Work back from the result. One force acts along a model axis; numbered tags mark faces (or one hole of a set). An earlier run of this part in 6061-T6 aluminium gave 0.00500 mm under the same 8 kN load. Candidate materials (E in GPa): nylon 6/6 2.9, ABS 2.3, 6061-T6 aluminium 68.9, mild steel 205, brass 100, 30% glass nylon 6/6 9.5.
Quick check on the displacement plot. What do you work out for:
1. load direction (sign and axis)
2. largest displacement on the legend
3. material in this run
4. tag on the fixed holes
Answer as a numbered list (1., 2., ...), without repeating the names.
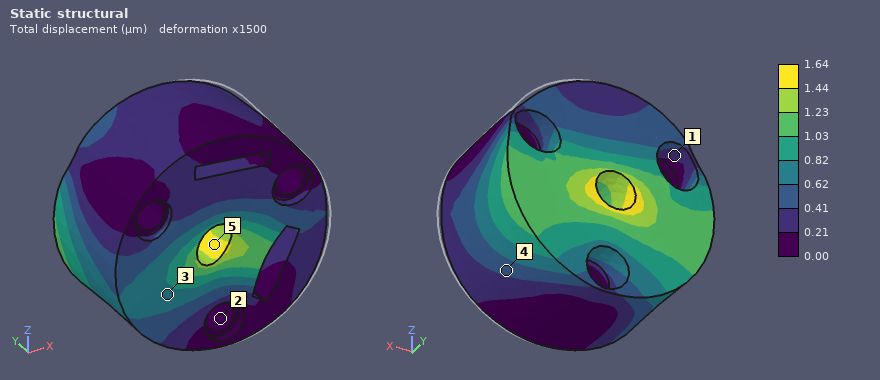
1. -X
2. 1.64 µm
3. mild steel
4. 2
